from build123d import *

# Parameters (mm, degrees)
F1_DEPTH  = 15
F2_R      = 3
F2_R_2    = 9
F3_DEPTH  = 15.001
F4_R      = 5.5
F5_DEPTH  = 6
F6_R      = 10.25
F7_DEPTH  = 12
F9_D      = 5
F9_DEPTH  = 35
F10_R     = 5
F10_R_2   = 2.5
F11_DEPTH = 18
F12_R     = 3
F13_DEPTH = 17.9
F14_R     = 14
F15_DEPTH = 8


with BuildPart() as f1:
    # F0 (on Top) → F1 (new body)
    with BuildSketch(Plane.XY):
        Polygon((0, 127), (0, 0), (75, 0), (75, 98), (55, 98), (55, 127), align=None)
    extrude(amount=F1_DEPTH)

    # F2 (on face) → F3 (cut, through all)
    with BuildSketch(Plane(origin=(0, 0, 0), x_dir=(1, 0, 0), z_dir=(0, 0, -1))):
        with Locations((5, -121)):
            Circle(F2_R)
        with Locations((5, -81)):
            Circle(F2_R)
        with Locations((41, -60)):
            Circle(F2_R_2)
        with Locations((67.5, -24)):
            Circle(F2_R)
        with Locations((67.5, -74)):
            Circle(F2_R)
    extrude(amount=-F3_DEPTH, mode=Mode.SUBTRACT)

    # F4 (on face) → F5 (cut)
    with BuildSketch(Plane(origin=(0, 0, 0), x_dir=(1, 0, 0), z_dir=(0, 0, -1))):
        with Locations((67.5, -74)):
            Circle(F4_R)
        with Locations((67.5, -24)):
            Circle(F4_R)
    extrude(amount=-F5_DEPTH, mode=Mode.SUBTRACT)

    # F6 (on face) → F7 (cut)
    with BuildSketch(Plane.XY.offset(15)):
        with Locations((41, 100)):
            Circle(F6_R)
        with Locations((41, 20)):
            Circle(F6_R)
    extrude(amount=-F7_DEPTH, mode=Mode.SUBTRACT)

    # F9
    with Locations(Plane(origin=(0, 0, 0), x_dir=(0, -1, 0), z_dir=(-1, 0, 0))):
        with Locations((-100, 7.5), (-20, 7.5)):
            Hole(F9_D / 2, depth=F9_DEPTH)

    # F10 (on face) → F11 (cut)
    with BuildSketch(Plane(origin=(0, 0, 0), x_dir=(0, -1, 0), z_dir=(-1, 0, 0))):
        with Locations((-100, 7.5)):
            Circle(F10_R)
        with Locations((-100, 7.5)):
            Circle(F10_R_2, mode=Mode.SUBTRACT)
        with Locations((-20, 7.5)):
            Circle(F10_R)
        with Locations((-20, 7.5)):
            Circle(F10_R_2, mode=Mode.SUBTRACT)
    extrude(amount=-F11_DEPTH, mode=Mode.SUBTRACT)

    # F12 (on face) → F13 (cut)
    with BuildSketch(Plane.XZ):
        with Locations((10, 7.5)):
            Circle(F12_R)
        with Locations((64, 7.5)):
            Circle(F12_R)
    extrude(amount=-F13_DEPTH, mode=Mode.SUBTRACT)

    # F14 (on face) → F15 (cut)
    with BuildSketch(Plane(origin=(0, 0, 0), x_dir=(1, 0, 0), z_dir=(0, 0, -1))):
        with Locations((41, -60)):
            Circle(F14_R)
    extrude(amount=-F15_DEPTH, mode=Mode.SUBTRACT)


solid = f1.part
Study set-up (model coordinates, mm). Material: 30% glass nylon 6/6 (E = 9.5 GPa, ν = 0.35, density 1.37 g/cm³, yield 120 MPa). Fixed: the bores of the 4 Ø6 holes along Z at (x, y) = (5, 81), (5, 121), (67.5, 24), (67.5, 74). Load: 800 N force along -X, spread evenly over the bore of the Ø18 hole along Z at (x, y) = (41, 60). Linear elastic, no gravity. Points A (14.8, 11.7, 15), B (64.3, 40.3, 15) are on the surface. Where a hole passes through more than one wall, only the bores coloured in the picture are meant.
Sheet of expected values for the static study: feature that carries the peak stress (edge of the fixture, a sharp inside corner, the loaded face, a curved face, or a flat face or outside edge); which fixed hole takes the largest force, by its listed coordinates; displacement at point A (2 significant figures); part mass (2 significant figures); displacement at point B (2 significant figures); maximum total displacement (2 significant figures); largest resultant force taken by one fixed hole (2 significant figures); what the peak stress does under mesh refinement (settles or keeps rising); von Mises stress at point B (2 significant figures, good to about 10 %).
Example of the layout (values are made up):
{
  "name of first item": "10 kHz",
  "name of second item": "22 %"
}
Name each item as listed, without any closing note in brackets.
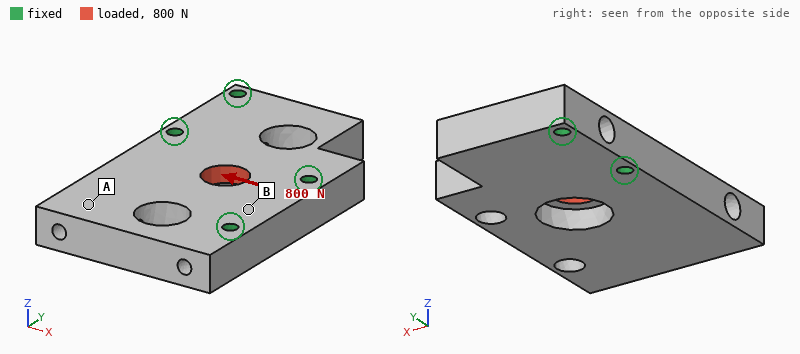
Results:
{
  "feature that carries the peak stress": "edge of the fixture",
  "which fixed hole takes the largest force, by its listed coordinates": "(67.5, 74)",
  "displacement at point A": "4.0 µm",
  "part mass": "150 g",
  "displacement at point B": "3.2 µm",
  "maximum total displacement": "7.7 µm",
  "largest resultant force taken by one fixed hole": "330 N",
  "what the peak stress does under mesh refinement": "keeps rising",
  "von Mises stress at point B": "0.89 MPa"
}
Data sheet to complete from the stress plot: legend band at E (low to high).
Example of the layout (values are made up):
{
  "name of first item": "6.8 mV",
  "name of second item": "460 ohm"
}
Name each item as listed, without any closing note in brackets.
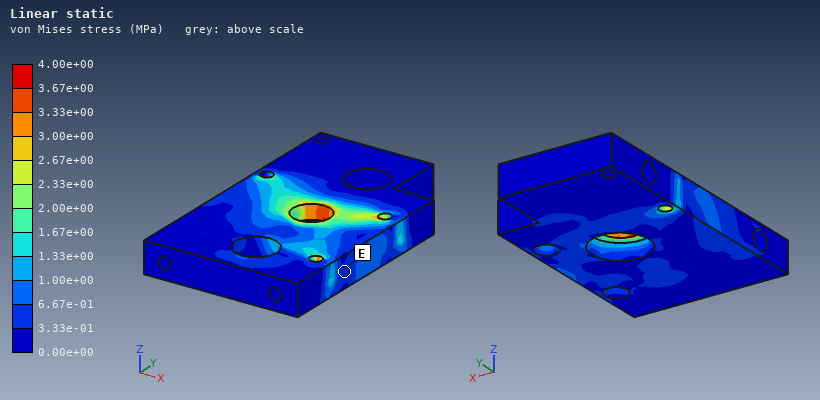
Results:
{
  "legend band at E": "3.33e-01 to 6.67e-01 MPa"
}
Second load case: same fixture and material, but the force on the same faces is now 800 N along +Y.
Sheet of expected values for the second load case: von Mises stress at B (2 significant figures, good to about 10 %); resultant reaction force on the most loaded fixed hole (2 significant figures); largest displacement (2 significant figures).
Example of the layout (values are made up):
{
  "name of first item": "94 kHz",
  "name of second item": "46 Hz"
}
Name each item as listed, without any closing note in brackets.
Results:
{
  "von Mises stress at B": "0.84 MPa",
  "resultant reaction force on the most loaded fixed hole": "280 N",
  "largest displacement": "10 µm"
}
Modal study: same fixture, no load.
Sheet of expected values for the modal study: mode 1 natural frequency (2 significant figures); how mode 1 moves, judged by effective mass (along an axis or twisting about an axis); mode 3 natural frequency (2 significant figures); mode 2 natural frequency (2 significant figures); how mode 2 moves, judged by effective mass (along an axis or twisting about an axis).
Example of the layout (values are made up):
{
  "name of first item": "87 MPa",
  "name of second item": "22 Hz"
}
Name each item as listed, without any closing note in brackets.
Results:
{
  "mode 1 natural frequency": "1700 Hz",
  "how mode 1 moves, judged by effective mass": "along Z",
  "mode 3 natural frequency": "4700 Hz",
  "mode 2 natural frequency": "3700 Hz",
  "how mode 2 moves, judged by effective mass": "along Z"
}
